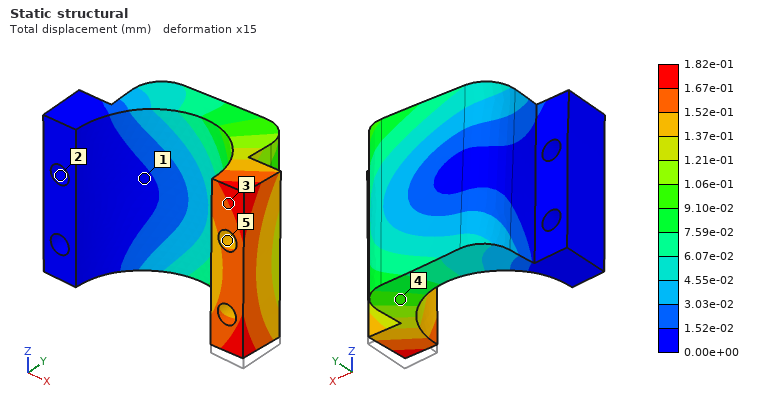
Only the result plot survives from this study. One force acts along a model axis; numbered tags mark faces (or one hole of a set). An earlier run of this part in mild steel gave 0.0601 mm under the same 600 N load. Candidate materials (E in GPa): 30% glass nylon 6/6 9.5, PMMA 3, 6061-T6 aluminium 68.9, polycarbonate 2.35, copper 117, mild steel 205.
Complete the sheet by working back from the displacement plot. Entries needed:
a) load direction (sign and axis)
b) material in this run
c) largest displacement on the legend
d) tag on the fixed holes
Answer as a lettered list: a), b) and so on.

a) +Z
b) 6061-T6 aluminium
c) 1.82e-01 mm
d) 2
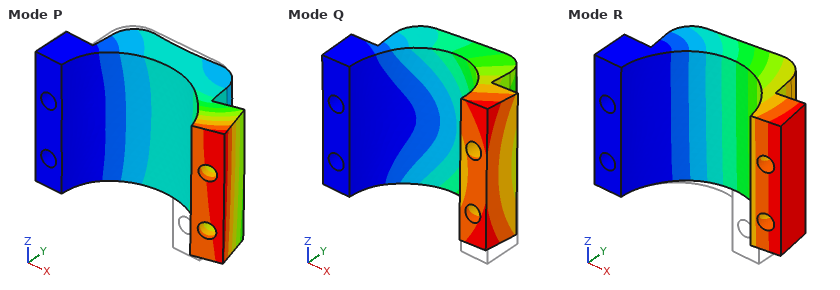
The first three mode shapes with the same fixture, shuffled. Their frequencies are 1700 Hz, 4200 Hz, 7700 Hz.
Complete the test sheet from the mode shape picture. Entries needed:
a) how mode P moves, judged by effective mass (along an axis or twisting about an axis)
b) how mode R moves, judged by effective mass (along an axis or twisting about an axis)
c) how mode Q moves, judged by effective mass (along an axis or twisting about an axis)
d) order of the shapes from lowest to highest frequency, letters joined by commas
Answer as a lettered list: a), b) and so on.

a) along X
b) along Y
c) along Z
d) R, Q, P
